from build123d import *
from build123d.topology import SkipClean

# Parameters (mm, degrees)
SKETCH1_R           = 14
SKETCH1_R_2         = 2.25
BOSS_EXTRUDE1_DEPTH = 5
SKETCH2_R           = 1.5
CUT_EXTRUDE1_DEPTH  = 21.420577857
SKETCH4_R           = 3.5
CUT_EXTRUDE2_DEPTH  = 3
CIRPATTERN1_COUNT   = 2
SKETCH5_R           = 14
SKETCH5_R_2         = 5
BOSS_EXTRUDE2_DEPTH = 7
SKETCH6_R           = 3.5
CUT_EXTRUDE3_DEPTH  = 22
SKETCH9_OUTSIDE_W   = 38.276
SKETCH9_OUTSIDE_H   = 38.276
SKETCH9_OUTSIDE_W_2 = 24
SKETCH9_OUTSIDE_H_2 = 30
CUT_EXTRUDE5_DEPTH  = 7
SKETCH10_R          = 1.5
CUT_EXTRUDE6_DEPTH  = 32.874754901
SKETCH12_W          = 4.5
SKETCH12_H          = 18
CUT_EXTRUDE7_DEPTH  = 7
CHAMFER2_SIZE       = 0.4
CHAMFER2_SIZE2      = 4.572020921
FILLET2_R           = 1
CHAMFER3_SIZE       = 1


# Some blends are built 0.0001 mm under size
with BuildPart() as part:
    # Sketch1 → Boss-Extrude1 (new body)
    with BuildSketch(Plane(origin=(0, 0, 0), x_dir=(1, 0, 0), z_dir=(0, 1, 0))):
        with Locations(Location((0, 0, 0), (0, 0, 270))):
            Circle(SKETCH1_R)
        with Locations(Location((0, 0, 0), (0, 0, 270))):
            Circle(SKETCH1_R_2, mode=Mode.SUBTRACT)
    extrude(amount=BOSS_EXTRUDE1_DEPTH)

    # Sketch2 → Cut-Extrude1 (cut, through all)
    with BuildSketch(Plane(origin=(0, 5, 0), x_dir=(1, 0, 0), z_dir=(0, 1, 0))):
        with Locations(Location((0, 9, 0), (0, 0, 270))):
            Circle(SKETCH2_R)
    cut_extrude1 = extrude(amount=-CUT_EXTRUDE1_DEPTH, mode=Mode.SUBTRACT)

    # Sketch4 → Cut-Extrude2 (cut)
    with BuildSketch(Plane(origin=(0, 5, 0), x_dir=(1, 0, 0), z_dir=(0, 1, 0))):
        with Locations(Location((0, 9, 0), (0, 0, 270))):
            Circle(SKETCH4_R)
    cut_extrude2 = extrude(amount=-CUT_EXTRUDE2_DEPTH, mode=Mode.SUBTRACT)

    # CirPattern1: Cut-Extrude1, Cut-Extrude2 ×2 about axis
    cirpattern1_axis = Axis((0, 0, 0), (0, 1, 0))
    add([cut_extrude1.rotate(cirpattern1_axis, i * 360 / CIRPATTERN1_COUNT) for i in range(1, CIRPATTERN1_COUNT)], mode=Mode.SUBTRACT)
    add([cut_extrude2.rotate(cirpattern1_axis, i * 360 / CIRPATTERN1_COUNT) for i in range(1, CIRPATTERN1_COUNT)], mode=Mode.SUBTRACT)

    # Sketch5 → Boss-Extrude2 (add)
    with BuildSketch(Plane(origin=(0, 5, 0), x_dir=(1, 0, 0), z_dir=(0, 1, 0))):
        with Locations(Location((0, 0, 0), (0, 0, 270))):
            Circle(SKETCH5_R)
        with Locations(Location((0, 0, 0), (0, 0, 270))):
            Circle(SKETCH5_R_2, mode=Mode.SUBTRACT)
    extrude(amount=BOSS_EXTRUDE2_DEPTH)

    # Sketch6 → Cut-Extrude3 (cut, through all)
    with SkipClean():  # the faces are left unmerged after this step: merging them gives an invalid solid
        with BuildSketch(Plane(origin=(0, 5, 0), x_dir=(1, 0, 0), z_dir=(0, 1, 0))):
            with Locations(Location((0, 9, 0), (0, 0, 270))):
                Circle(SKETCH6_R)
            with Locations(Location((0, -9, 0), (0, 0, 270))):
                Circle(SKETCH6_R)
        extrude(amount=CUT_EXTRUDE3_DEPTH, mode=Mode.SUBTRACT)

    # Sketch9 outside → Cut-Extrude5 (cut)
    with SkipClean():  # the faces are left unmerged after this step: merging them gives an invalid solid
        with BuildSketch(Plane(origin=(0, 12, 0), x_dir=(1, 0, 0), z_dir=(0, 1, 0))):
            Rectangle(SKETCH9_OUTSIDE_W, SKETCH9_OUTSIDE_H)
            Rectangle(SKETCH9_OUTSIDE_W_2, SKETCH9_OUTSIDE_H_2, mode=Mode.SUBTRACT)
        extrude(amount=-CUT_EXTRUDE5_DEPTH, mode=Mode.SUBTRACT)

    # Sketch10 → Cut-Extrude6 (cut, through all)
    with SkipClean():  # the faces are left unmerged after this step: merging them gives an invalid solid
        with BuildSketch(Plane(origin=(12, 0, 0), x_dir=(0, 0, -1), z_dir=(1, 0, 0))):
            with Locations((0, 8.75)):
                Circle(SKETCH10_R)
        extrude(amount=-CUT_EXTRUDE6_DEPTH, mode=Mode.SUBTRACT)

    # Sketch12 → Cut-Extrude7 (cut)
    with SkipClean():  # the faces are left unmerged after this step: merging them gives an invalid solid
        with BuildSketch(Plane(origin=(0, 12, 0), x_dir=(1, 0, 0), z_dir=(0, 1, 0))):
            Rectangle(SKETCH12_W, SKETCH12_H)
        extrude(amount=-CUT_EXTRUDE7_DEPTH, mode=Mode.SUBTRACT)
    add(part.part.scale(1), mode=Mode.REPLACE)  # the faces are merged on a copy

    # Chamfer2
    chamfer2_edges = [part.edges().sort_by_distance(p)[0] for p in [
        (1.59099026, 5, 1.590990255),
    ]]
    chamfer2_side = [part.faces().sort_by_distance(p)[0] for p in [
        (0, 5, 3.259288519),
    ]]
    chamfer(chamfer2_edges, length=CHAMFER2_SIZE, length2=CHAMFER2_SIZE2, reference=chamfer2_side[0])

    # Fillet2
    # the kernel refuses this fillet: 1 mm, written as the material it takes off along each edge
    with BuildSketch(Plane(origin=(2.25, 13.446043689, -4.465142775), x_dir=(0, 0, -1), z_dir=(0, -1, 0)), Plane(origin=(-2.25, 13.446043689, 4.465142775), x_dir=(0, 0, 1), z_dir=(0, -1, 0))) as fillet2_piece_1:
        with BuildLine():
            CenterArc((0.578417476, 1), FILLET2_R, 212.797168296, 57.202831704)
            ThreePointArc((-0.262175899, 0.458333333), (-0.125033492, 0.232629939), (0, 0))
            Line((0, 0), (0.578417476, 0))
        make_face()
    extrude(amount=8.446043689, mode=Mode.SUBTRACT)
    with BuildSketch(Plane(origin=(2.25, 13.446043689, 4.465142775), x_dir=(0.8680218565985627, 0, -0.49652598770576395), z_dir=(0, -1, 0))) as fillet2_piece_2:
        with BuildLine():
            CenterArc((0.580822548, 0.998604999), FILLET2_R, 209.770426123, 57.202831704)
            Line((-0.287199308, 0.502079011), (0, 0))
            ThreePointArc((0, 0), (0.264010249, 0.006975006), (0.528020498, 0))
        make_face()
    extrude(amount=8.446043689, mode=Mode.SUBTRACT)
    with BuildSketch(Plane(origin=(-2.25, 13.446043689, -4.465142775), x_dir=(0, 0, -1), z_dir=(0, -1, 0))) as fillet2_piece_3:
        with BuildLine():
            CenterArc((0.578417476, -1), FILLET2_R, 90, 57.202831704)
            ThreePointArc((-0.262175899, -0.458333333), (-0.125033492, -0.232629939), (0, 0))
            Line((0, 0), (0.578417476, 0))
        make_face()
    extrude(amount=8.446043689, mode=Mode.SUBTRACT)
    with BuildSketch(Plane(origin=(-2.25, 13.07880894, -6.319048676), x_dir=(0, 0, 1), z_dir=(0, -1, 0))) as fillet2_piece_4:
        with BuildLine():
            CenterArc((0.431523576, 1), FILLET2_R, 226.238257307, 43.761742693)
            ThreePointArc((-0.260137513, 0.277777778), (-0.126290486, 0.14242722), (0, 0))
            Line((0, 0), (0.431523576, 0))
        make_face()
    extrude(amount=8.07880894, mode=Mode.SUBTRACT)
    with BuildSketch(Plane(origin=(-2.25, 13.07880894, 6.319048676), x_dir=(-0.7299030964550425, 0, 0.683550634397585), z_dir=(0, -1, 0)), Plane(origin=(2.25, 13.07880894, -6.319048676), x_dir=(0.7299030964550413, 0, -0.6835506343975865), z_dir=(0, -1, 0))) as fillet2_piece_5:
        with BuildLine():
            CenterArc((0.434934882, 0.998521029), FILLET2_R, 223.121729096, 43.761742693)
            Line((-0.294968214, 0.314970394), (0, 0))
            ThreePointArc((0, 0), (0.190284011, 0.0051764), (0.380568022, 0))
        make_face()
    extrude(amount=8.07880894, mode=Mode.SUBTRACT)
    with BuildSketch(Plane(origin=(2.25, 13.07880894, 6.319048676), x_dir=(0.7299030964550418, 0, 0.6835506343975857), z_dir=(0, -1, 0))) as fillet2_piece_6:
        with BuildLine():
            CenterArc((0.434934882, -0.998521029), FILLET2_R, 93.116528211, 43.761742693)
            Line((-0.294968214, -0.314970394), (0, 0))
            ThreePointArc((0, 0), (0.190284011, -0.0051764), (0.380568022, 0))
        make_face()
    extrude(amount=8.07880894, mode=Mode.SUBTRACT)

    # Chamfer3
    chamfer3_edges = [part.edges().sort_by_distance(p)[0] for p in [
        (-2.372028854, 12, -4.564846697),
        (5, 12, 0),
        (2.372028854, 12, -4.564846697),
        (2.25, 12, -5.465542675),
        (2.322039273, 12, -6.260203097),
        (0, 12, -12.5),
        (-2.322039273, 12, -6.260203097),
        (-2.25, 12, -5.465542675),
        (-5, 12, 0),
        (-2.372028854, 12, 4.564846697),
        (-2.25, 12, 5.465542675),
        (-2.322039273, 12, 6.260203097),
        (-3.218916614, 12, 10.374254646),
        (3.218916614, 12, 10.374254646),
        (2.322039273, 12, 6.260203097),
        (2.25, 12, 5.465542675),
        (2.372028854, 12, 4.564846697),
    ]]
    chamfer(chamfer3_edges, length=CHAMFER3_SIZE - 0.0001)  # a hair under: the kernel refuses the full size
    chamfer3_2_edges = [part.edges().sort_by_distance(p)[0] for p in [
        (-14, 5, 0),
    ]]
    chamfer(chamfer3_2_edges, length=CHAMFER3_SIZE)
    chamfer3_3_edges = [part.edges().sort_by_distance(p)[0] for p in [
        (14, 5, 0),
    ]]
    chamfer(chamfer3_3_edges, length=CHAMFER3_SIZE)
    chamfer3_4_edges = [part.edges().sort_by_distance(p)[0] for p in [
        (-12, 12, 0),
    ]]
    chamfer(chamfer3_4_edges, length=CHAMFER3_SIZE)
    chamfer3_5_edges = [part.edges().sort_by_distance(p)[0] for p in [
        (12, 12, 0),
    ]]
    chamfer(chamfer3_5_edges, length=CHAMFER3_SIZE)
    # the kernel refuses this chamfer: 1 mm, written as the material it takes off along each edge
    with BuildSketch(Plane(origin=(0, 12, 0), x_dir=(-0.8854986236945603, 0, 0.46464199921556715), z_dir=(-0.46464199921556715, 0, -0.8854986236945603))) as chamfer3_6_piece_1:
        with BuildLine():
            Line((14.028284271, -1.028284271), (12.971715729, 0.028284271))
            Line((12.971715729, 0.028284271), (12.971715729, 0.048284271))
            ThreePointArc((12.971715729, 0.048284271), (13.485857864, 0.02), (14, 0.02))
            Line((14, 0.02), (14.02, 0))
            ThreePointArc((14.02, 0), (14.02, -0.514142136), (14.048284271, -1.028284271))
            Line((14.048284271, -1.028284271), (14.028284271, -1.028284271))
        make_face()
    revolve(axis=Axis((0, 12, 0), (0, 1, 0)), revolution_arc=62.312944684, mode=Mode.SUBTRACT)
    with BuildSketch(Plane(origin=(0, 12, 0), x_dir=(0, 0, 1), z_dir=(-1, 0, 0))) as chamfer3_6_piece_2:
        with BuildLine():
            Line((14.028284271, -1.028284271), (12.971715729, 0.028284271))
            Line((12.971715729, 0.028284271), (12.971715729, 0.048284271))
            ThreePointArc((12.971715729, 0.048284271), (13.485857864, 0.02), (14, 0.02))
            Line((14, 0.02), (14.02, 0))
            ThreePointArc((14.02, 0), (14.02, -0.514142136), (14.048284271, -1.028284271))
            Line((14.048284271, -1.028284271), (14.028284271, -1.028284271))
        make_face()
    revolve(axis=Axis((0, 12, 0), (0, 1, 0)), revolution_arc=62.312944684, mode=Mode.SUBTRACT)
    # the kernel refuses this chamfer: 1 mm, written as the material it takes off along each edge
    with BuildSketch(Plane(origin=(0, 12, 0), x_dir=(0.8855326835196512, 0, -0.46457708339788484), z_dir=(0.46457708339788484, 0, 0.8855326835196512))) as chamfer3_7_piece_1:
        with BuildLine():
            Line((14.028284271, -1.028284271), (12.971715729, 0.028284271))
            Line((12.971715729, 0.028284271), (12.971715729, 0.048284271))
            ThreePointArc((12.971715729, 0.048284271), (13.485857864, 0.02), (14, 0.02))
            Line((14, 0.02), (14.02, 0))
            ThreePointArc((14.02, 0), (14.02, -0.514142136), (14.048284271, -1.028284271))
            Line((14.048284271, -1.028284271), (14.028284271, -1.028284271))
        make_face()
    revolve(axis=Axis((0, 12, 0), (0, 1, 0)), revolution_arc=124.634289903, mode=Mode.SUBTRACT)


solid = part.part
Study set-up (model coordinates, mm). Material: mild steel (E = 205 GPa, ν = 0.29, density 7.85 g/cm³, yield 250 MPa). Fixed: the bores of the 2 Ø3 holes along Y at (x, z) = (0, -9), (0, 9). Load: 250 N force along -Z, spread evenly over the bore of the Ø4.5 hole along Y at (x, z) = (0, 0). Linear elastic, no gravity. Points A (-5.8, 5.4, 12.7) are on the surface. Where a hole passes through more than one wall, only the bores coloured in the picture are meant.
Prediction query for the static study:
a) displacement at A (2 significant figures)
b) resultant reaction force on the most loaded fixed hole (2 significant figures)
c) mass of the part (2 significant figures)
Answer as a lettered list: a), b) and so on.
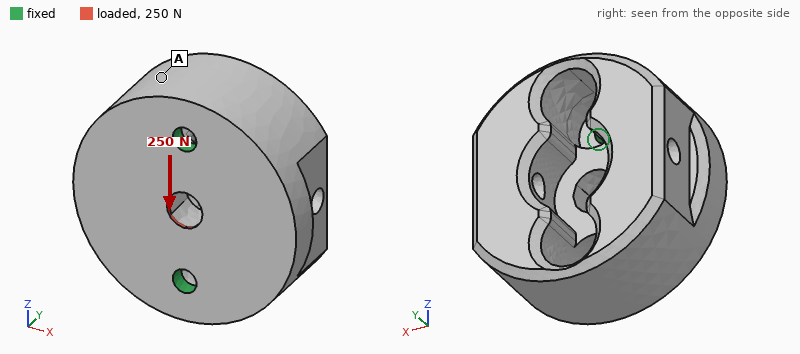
a) 0.10 µm
b) 130 N
c) 43 g
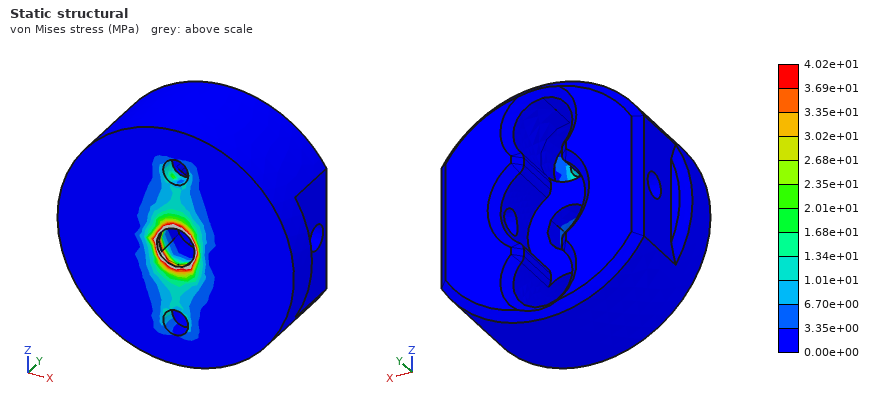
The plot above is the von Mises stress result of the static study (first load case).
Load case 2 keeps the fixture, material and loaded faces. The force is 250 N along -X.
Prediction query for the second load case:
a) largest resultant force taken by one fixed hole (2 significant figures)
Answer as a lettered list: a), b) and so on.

a) 130 N
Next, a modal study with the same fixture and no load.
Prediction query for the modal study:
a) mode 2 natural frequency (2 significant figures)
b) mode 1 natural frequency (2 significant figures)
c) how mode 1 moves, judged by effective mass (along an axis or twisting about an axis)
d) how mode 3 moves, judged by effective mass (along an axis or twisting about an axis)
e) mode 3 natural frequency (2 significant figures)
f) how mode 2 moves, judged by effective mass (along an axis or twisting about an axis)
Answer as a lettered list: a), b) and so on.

a) 18 kHz
b) 5600 Hz
c) along X
d) along Z
e) 21 kHz
f) along Y
